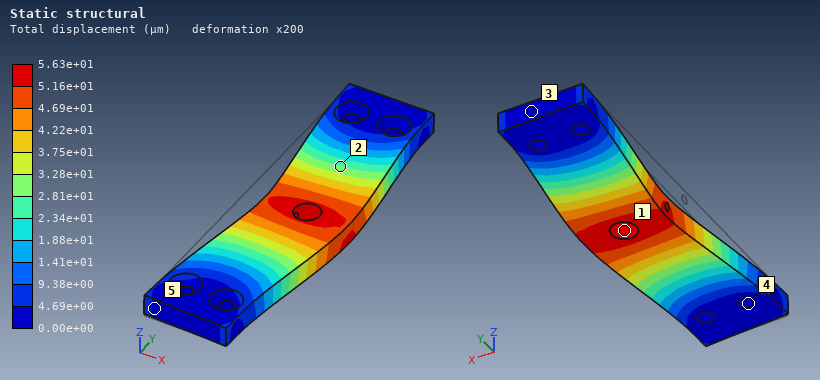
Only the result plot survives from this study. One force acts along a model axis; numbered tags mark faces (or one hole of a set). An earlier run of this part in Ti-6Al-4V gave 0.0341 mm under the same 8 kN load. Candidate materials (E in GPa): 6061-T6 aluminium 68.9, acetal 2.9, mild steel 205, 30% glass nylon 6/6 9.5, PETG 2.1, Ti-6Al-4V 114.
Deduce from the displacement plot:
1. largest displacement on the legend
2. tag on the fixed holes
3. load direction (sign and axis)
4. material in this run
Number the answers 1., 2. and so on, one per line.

1. 5.63e+01 µm
2. 4
3. +X
4. 6061-T6 aluminium
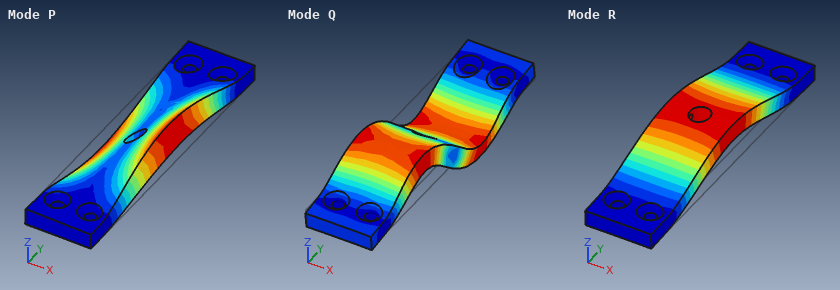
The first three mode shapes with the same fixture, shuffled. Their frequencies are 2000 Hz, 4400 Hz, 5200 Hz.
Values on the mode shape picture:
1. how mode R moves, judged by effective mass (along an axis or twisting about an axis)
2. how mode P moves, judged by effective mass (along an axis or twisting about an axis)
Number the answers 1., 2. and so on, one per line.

1. along Z
2. twisting about Y
